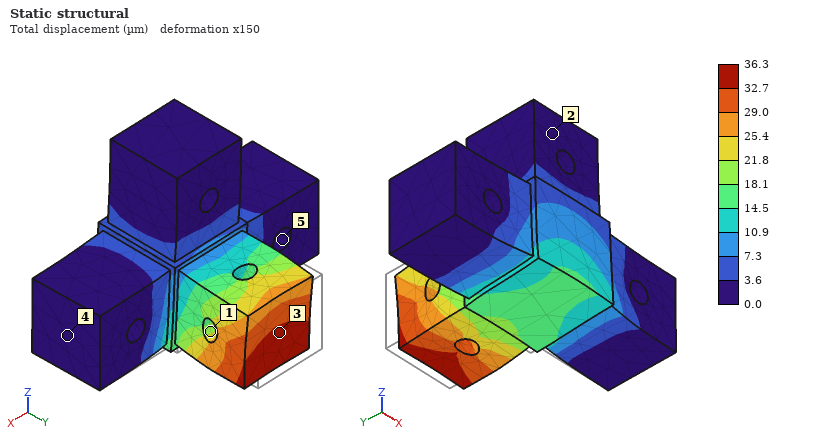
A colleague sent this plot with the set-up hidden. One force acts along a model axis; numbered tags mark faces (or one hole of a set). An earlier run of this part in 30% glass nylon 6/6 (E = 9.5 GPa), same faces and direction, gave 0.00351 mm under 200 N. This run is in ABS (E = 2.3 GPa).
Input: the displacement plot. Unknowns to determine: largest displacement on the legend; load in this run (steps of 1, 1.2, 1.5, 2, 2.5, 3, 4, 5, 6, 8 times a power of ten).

36.3 µm
500 N
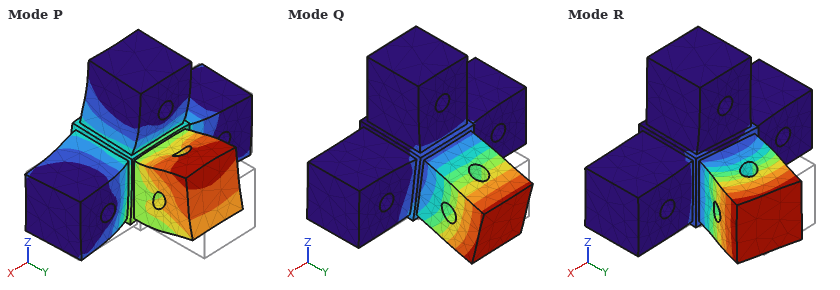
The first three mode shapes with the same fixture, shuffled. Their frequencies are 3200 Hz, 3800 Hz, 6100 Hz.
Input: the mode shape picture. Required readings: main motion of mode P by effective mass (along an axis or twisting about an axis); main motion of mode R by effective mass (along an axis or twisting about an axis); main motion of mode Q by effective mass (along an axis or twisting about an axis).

along Y
along X
along Z
